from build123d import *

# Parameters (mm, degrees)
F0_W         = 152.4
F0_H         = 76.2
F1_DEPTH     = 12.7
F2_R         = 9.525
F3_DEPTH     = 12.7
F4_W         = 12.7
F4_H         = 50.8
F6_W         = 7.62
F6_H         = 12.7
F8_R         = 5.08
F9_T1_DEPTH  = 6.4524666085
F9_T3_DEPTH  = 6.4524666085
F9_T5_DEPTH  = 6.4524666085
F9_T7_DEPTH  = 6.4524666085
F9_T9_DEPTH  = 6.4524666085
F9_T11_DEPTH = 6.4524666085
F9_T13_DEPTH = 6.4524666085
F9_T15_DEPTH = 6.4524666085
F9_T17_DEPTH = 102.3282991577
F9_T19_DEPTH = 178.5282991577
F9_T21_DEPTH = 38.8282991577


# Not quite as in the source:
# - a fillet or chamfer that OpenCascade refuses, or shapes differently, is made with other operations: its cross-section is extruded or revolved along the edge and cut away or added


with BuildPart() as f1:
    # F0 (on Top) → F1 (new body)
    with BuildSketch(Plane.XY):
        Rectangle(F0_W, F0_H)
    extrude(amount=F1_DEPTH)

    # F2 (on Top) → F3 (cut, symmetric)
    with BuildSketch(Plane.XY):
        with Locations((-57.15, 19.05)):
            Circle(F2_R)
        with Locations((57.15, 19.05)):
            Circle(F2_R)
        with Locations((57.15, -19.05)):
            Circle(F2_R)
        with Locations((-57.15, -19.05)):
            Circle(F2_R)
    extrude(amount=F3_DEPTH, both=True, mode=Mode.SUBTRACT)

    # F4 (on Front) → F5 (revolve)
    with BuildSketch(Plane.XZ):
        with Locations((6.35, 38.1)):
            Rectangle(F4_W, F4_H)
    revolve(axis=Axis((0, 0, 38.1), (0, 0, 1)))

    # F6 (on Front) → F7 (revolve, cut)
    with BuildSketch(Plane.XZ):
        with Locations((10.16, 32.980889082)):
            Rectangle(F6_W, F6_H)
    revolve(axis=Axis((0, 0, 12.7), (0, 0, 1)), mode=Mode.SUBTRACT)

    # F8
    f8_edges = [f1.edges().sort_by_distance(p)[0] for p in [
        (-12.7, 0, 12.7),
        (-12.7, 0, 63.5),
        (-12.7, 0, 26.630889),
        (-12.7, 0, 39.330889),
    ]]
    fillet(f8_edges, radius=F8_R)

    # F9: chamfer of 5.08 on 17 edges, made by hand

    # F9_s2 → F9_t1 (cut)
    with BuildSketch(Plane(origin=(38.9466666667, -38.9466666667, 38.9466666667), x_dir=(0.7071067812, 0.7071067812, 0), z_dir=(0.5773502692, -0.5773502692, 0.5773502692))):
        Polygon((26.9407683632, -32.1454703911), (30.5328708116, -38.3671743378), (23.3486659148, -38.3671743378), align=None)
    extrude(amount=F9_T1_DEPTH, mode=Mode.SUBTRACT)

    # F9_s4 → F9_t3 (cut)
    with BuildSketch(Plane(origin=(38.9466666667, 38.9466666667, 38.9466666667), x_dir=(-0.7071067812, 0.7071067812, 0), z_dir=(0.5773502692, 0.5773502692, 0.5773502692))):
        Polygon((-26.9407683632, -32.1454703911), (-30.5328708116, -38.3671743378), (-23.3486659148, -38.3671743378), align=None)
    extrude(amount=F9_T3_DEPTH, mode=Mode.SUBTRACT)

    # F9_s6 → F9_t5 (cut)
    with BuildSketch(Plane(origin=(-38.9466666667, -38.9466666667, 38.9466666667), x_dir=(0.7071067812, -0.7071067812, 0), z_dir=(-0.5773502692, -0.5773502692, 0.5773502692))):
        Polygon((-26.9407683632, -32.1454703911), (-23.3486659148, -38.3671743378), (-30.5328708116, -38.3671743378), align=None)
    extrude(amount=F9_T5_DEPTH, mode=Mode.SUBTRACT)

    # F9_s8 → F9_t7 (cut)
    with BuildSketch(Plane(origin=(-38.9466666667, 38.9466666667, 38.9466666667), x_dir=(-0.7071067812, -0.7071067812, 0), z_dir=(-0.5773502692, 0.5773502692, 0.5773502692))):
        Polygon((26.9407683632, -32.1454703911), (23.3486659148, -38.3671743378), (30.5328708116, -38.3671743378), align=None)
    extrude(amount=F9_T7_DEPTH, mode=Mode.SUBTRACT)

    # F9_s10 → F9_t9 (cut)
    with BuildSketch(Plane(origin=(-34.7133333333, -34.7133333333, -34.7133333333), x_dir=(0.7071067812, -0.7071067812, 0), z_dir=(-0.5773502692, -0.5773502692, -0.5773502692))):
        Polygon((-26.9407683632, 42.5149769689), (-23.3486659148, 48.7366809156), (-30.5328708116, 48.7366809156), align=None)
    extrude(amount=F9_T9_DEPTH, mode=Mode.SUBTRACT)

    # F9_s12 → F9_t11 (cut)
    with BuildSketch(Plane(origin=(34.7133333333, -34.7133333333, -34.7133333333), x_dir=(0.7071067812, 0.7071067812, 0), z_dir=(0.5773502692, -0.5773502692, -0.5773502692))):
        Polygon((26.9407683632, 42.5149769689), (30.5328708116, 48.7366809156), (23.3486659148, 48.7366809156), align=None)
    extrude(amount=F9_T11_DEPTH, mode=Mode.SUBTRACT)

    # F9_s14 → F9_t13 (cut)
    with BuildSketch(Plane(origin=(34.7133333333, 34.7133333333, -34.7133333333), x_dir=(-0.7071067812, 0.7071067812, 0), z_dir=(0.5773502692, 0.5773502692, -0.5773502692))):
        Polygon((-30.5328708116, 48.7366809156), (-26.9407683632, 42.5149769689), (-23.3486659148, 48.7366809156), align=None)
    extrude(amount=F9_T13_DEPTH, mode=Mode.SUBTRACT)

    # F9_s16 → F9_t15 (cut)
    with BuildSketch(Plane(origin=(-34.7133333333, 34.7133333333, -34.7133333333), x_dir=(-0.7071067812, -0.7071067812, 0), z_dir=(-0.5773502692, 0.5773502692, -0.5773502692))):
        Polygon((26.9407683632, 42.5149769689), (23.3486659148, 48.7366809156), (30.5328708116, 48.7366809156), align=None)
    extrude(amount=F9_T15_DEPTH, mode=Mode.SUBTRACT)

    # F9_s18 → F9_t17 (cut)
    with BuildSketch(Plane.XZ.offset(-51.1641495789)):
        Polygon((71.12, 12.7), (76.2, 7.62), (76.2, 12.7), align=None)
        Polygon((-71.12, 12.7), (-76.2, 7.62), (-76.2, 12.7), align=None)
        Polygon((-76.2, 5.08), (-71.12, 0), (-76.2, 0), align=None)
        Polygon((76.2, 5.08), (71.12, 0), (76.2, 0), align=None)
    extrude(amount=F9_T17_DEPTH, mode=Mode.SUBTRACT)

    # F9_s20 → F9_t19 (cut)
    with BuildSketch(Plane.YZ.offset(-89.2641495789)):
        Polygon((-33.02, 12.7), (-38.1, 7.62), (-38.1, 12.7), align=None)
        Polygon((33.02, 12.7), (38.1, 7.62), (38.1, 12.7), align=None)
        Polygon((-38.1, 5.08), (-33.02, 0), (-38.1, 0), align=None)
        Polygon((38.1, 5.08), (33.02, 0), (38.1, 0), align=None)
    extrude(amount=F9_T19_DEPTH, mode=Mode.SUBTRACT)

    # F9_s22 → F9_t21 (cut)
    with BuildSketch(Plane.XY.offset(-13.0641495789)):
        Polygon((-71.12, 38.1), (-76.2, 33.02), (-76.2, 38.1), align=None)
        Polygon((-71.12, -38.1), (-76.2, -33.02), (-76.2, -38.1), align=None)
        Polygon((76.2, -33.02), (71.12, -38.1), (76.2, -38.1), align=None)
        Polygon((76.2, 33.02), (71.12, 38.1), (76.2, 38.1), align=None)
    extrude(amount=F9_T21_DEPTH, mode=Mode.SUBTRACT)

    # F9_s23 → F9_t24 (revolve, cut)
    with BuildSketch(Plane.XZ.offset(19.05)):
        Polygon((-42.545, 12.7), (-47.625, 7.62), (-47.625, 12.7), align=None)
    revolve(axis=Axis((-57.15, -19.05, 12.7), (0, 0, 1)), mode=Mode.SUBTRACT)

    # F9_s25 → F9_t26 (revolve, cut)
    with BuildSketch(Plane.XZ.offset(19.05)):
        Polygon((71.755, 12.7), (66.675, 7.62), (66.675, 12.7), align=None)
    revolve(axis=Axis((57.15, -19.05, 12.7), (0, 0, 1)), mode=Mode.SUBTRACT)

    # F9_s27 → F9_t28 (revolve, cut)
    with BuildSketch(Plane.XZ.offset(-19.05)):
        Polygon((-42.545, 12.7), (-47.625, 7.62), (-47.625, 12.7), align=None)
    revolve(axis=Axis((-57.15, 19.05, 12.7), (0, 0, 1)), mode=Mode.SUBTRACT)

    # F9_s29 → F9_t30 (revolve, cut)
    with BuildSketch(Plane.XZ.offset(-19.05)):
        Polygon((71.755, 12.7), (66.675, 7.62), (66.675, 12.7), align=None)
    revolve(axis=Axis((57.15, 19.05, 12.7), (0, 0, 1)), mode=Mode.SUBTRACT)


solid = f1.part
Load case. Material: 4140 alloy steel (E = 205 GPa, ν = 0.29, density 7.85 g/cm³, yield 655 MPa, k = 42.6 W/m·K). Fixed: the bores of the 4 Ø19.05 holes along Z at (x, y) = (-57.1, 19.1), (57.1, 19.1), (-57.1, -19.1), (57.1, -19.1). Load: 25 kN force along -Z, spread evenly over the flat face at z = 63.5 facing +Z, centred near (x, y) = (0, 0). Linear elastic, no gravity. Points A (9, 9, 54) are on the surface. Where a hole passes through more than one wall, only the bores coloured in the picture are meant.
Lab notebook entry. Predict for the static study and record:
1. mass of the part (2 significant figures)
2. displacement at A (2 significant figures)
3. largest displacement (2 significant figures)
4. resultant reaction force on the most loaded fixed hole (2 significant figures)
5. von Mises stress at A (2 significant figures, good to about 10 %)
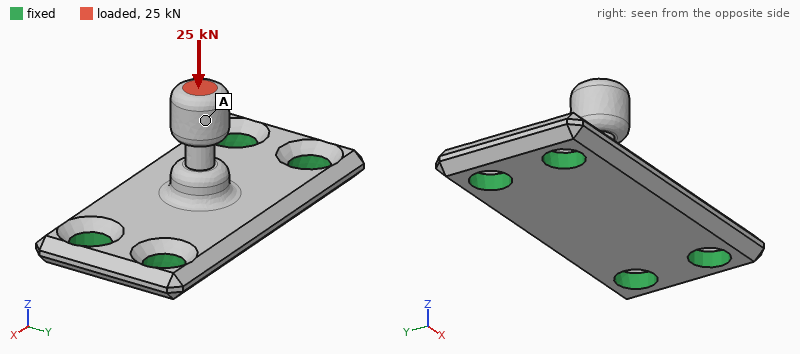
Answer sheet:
1.1 kg
85 µm
92 µm
8.0 kN
32 MPa
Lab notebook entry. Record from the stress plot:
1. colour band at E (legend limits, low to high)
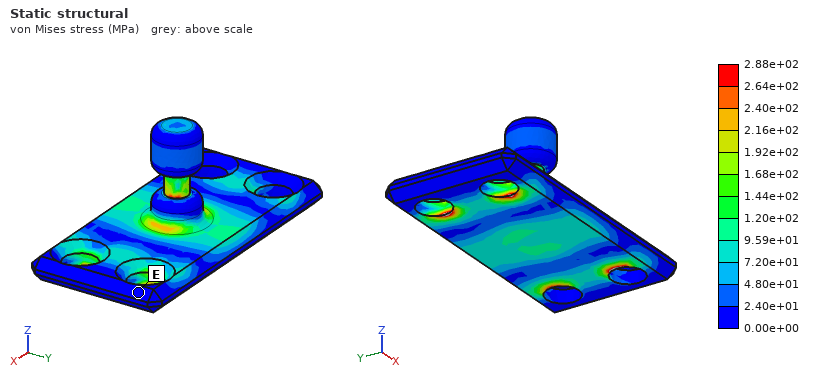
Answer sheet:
0.00e+00 to 2.40e+01 MPa
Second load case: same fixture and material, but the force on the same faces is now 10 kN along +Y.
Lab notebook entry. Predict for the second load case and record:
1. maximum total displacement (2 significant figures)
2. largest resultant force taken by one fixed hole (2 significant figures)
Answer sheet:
0.90 mm
8.6 kN
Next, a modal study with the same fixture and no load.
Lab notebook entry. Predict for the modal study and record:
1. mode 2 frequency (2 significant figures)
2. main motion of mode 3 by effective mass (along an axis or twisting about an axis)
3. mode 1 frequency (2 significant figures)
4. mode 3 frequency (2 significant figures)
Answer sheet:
2700 Hz
along Z
2500 Hz
4500 Hz
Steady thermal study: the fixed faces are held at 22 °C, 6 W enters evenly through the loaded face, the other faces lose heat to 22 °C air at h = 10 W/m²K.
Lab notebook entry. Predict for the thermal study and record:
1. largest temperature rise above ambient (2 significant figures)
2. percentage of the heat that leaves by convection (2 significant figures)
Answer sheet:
32 K
17 %
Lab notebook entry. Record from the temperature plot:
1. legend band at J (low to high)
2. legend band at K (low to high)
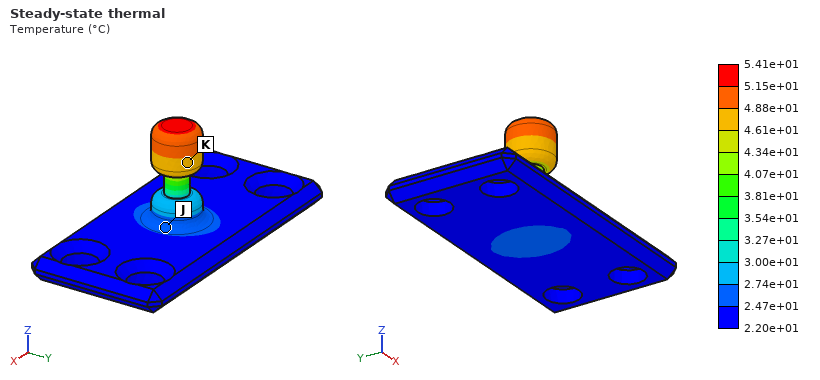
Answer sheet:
2.47e+01 to 2.74e+01 °C
4.61e+01 to 4.88e+01 °C
